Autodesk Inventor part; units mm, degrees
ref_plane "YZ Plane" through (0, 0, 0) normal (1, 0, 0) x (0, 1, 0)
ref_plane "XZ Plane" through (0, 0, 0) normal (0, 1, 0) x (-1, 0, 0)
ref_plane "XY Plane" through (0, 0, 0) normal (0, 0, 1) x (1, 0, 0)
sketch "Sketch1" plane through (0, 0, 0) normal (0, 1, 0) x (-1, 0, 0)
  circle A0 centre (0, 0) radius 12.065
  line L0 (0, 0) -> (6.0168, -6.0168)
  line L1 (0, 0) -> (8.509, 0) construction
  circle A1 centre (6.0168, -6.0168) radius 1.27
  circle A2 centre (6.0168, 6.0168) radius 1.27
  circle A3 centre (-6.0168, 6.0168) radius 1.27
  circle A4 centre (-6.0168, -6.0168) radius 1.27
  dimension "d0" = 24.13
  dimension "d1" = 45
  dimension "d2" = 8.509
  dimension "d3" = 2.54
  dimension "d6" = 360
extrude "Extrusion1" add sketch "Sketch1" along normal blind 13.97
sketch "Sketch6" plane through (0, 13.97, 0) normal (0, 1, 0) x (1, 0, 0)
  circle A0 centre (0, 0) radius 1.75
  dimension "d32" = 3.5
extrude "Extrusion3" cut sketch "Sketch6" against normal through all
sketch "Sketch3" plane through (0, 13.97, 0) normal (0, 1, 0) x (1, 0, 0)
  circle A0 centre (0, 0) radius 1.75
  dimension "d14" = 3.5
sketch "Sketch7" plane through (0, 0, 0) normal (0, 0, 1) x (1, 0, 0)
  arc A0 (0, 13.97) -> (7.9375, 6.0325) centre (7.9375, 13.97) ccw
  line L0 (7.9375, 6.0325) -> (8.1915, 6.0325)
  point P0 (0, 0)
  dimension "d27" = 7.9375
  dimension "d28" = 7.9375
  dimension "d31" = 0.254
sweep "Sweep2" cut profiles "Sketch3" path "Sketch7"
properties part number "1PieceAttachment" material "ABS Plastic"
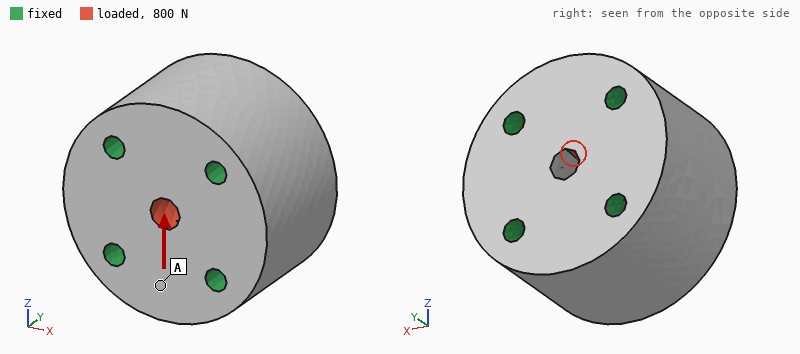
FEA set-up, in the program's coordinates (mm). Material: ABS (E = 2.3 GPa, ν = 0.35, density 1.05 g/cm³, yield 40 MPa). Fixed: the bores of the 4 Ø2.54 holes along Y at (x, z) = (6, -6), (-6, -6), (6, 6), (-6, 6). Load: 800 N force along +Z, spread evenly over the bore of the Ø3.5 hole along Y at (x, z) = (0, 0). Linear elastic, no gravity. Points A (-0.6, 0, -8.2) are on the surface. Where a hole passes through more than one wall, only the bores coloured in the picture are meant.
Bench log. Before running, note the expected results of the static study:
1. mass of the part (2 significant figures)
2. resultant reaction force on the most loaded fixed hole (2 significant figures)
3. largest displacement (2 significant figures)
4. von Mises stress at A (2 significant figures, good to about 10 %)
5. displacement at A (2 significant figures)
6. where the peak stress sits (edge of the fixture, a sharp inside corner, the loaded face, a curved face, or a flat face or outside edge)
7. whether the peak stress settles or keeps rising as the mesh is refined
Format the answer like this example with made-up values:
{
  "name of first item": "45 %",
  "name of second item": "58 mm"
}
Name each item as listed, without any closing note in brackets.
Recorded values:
{
  "mass of the part": "6.2 g",
  "resultant reaction force on the most loaded fixed hole": "240 N",
  "largest displacement": "16 µm",
  "von Mises stress at A": "1.4 MPa",
  "displacement at A": "7.3 µm",
  "where the peak stress sits": "a sharp inside corner",
  "whether the peak stress settles or keeps rising as the mesh is refined": "keeps rising"
}
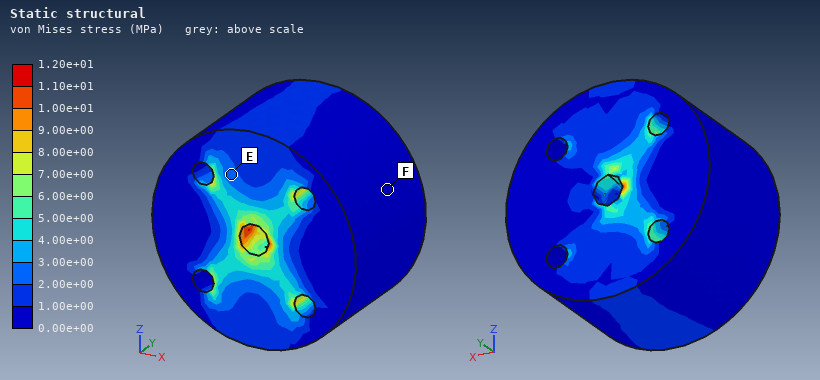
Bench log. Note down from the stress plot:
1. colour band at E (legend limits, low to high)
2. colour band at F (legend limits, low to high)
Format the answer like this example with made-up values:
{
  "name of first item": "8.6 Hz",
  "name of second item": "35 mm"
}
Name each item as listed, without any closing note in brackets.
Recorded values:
{
  "colour band at E": "2.00e+00 to 3.00e+00 MPa",
  "colour band at F": "0.00e+00 to 1.00e+00 MPa"
}
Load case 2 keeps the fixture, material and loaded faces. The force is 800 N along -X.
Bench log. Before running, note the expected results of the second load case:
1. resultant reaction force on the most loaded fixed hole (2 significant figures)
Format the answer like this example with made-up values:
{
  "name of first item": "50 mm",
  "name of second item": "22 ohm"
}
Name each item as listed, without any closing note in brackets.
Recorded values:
{
  "resultant reaction force on the most loaded fixed hole": "230 N"
}
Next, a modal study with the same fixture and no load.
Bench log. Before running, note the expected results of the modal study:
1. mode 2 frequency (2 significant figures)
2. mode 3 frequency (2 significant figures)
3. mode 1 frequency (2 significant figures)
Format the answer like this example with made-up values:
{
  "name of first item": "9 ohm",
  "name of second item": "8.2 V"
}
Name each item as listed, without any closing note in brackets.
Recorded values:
{
  "mode 2 frequency": "30 kHz",
  "mode 3 frequency": "30 kHz",
  "mode 1 frequency": "30 kHz"
}
